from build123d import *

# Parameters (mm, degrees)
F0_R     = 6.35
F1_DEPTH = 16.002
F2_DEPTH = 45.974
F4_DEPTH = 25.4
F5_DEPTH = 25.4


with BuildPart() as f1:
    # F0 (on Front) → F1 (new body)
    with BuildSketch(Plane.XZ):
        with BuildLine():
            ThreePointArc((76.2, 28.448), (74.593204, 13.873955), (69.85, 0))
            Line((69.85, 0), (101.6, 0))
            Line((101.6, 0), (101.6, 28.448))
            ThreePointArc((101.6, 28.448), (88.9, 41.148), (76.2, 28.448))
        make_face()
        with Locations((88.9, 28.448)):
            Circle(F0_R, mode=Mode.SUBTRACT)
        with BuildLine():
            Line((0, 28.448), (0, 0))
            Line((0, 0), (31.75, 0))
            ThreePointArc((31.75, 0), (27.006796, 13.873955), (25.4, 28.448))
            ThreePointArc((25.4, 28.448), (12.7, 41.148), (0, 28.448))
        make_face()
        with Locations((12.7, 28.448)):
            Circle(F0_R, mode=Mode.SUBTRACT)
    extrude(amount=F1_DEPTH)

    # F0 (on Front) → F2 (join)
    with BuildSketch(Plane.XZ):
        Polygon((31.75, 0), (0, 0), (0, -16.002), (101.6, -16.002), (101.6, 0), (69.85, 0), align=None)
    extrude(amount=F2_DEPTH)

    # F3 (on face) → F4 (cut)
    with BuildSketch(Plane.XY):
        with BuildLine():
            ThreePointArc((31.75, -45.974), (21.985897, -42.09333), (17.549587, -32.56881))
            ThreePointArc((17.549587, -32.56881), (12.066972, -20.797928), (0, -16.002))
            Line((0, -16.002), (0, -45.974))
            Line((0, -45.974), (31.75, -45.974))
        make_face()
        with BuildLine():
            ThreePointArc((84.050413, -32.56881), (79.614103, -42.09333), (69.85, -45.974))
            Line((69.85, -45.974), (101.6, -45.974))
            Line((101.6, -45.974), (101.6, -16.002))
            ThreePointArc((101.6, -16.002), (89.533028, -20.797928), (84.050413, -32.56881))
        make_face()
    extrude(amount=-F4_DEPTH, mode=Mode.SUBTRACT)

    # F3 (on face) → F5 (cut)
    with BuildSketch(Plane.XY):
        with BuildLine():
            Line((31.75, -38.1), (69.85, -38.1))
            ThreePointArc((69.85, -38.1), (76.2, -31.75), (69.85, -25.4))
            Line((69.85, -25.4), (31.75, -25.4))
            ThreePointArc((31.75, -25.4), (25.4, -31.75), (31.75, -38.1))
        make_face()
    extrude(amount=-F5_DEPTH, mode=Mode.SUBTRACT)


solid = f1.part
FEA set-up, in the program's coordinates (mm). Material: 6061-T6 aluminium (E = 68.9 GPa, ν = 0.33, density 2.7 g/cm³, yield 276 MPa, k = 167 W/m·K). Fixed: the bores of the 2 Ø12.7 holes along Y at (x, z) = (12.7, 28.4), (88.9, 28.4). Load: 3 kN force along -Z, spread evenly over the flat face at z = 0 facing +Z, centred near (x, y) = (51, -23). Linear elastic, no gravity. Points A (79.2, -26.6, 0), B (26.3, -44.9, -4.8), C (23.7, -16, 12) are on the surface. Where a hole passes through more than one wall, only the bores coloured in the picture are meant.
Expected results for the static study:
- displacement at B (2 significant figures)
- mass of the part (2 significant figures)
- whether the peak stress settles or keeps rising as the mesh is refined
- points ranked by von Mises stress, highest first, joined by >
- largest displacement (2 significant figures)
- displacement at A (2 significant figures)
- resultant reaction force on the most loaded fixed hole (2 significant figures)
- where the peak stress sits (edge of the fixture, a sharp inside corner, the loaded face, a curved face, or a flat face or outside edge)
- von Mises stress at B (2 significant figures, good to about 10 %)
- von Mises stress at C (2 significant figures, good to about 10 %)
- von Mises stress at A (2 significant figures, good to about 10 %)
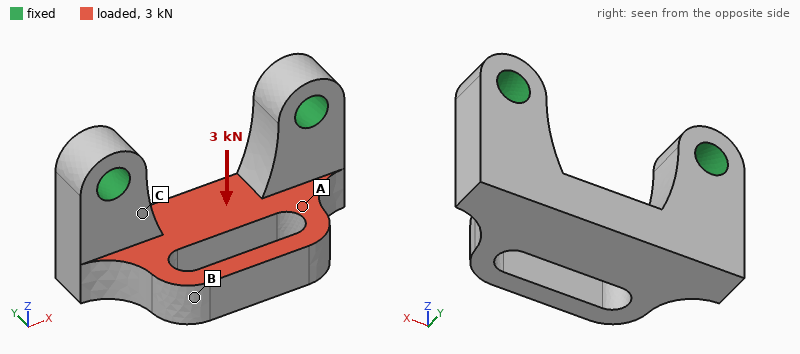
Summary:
59 µm
210 g
keeps rising
C > A > B
72 µm
27 µm
1.6 kN
edge of the fixture
5.2 MPa
25 MPa
15 MPa
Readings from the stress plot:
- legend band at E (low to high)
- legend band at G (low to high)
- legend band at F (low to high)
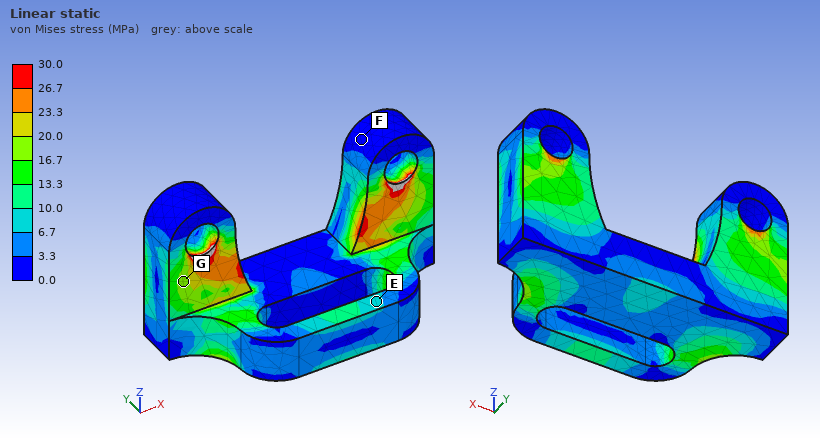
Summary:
6.7 to 10.0 MPa
16.7 to 20.0 MPa
0.0 to 3.3 MPa
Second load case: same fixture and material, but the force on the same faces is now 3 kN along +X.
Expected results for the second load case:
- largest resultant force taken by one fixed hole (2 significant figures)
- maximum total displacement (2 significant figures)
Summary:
1.6 kN
31 µm
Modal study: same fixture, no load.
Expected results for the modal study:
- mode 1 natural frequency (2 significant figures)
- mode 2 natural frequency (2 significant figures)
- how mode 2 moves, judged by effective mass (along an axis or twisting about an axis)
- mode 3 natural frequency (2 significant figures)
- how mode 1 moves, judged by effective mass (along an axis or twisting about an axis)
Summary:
3200 Hz
5600 Hz
along X
7100 Hz
along Y
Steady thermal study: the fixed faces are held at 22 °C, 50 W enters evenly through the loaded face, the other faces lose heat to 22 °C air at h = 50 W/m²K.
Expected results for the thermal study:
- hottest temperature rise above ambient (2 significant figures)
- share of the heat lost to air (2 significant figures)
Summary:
19 K
13 %
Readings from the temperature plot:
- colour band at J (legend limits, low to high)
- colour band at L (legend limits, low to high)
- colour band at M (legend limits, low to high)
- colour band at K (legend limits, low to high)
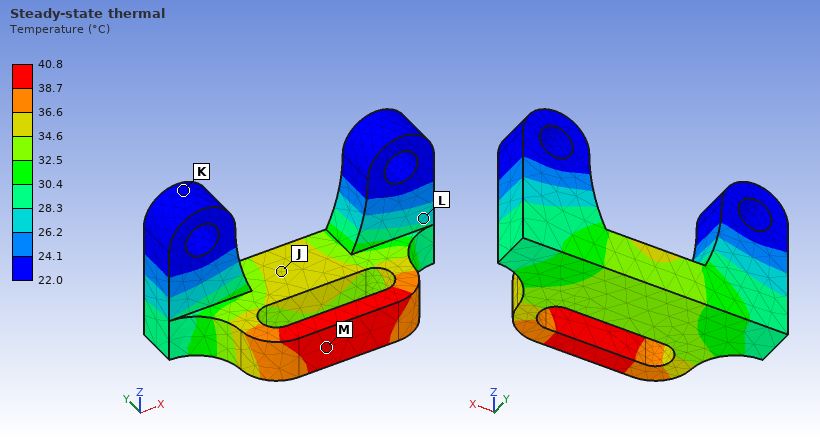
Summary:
34.6 to 36.6 °C
26.2 to 28.3 °C
38.7 to 40.8 °C
22.0 to 24.1 °C
